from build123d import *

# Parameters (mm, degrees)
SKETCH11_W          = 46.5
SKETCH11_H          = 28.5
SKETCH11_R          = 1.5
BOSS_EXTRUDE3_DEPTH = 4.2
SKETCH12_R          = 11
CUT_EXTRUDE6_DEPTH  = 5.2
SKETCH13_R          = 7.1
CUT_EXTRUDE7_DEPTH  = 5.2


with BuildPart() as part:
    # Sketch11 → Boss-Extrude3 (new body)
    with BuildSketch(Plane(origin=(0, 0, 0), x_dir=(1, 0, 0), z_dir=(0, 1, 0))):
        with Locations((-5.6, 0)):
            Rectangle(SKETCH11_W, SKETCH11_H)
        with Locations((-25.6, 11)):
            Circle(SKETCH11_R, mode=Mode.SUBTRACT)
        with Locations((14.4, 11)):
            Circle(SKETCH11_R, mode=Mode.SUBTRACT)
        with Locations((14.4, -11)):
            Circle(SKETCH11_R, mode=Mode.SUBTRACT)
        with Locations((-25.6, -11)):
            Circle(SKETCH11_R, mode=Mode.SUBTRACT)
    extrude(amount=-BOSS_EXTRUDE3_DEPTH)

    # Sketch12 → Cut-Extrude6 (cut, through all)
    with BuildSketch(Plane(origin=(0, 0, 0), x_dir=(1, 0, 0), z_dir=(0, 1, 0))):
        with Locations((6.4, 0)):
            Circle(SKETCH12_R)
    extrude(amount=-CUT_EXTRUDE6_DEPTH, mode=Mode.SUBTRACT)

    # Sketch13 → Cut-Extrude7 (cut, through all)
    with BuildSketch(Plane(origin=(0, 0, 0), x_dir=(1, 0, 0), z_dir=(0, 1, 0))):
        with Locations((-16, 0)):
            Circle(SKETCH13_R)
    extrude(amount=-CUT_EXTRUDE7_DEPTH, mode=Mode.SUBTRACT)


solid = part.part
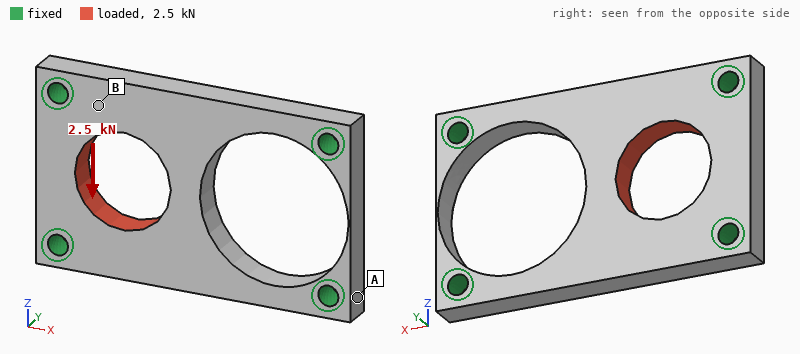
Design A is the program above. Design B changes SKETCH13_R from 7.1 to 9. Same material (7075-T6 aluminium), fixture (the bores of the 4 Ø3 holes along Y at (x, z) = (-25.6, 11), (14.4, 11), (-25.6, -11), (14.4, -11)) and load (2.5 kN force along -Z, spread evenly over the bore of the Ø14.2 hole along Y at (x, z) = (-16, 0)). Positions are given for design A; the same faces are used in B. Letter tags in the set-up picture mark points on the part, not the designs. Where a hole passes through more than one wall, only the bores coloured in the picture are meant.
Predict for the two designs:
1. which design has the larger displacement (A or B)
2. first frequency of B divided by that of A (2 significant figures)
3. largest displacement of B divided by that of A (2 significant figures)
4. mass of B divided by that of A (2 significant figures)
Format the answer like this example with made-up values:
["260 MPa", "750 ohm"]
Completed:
["B", "1.0", "1.5", "0.87"]
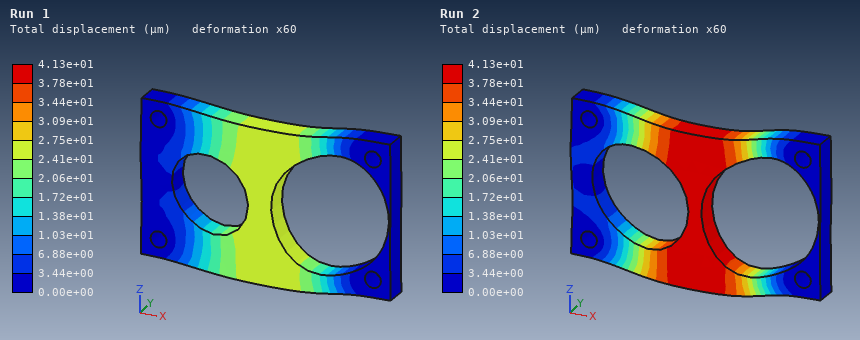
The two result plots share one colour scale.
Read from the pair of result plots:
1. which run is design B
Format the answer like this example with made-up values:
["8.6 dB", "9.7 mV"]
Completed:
["Run 2"]
